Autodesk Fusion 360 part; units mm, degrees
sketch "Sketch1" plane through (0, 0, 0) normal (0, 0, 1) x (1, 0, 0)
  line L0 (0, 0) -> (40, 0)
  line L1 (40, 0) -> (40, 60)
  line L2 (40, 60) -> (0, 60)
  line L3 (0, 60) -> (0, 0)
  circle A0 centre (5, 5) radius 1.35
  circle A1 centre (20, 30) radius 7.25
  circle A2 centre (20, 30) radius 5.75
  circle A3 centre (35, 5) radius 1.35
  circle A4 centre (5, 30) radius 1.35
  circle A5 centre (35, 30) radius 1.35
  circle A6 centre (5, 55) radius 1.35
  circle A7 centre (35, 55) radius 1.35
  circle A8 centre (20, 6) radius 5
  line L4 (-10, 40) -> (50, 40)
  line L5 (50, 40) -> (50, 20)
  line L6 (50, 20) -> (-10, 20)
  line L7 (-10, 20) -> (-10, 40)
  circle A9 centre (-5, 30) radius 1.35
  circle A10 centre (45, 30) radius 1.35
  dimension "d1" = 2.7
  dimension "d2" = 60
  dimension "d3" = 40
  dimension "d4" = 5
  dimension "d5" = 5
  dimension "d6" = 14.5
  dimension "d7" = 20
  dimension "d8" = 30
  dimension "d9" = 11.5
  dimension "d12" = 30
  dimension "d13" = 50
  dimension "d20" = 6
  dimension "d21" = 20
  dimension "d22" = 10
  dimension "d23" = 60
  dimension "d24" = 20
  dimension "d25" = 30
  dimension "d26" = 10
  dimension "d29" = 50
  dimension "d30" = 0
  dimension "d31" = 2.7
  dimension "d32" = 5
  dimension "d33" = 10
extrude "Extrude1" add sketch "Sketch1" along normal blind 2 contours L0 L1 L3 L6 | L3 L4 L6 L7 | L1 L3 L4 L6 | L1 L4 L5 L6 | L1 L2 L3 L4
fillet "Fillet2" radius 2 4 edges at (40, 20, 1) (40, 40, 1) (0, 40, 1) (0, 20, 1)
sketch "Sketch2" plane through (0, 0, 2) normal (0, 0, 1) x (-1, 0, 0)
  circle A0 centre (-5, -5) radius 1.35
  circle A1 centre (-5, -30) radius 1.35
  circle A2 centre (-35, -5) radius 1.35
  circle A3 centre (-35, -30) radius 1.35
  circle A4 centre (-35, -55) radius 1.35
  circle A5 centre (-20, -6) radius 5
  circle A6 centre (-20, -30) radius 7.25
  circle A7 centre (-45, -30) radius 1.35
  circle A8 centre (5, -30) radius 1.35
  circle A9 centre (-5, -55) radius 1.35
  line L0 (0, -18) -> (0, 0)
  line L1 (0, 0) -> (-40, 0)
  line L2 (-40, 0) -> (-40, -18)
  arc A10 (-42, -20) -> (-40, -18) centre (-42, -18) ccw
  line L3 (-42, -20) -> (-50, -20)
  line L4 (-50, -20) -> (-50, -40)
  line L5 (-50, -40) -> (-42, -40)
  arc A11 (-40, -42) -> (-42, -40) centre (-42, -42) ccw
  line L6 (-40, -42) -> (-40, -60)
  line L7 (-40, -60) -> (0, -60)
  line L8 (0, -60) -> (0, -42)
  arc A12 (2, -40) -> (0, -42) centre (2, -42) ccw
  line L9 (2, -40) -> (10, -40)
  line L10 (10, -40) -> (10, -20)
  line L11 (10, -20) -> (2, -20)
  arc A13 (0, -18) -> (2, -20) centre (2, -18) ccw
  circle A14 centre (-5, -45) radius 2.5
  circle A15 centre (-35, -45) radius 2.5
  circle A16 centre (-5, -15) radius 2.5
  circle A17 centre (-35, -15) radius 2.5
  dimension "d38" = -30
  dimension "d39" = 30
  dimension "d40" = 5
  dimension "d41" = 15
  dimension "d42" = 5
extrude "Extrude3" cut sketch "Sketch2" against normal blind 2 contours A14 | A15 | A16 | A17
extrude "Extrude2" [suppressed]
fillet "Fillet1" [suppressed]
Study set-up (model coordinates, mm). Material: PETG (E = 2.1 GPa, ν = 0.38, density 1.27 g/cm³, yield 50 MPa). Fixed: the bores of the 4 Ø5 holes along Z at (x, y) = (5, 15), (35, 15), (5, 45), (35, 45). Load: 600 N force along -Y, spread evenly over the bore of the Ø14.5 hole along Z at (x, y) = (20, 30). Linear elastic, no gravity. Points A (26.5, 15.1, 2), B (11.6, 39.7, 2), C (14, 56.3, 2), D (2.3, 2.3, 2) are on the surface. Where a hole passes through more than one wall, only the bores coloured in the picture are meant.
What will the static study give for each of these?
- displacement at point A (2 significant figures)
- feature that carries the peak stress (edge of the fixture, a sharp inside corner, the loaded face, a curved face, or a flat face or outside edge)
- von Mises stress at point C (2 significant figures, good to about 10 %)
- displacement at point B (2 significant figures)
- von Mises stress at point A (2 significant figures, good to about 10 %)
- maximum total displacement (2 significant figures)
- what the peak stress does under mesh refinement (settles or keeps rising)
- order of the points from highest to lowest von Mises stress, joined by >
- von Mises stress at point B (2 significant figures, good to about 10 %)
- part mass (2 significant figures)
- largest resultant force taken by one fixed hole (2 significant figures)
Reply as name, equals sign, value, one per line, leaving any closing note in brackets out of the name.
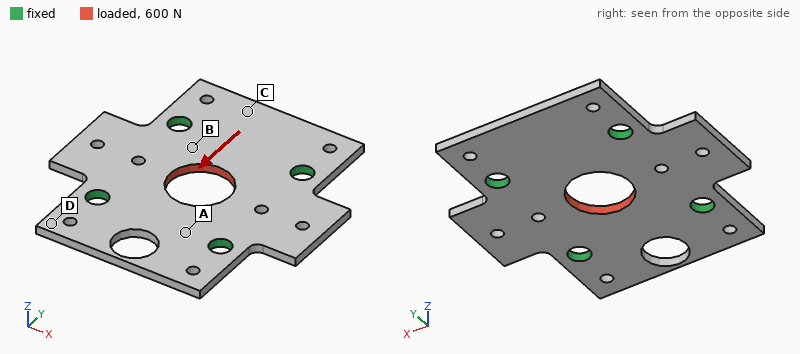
displacement at point A = 36 µm
feature that carries the peak stress = edge of the fixture
von Mises stress at point C = 2.3 MPa
displacement at point B = 29 µm
von Mises stress at point A = 4.6 MPa
maximum total displacement = 68 µm
what the peak stress does under mesh refinement = keeps rising
order of the points from highest to lowest von Mises stress, joined by > = B > A > C > D
von Mises stress at point B = 6.3 MPa
part mass = 6.2 g
largest resultant force taken by one fixed hole = 160 N
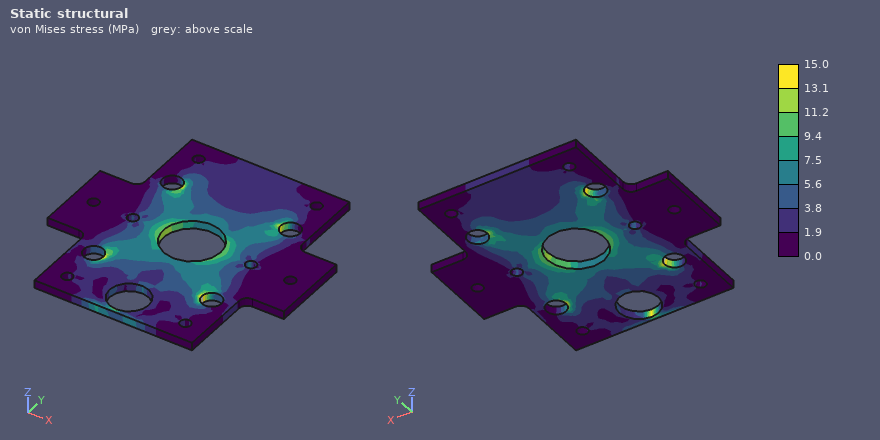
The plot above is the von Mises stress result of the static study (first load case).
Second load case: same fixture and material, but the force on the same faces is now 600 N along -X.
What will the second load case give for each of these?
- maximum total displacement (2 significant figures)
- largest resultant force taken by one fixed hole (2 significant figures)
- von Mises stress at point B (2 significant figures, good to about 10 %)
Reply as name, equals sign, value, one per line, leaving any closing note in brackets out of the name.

maximum total displacement = 67 µm
largest resultant force taken by one fixed hole = 160 N
von Mises stress at point B = 6.5 MPa
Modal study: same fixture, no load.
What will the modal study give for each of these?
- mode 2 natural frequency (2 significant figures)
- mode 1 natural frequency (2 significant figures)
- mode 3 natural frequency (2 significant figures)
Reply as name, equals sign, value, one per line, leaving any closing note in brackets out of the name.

mode 2 natural frequency = 1600 Hz
mode 1 natural frequency = 1600 Hz
mode 3 natural frequency = 1800 Hz
